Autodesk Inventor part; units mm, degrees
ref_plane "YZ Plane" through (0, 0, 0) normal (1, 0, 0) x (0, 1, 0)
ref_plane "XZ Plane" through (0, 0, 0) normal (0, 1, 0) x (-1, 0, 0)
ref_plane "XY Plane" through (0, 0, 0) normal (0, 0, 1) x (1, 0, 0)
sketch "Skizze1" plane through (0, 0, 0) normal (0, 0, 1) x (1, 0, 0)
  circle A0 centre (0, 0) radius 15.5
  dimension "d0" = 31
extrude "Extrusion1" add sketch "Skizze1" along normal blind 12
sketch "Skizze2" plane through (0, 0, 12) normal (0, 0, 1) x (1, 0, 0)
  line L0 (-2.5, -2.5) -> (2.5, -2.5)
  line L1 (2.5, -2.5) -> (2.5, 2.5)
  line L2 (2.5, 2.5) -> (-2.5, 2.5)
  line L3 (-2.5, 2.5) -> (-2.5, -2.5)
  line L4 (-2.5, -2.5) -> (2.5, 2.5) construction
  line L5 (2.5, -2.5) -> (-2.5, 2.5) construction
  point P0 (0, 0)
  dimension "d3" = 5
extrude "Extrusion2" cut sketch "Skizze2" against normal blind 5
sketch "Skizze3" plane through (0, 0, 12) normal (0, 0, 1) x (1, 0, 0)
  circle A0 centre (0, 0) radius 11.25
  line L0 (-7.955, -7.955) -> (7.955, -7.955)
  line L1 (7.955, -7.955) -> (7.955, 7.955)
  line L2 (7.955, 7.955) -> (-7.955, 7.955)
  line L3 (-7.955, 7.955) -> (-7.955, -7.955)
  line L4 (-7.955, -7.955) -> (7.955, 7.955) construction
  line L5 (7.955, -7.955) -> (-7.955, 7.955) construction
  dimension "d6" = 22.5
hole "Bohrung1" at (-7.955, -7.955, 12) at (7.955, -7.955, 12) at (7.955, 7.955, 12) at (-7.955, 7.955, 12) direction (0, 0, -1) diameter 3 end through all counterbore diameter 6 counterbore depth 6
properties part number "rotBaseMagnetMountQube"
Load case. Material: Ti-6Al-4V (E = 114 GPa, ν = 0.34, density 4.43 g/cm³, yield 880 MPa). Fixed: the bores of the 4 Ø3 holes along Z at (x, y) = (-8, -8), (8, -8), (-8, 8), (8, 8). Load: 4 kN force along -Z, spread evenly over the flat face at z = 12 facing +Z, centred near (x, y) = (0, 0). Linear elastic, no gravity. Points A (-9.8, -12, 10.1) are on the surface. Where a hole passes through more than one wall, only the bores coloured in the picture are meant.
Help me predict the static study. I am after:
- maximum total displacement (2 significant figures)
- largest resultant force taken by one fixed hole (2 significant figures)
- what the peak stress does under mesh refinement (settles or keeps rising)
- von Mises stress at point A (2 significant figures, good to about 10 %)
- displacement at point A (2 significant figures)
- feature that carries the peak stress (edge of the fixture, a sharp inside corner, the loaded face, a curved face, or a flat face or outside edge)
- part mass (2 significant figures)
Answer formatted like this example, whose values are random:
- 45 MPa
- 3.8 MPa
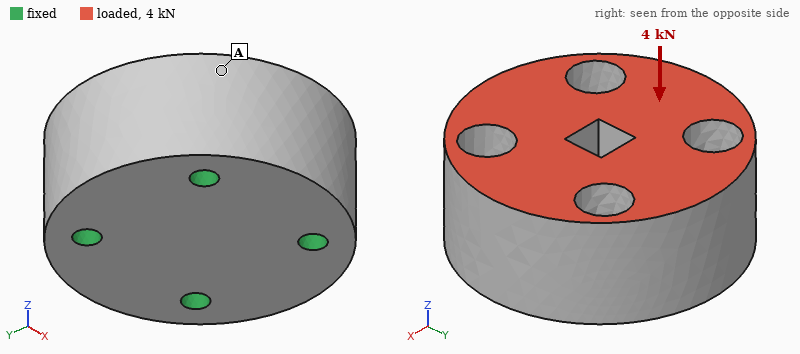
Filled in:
- 1.7 µm
- 1.0 kN
- keeps rising
- 9.1 MPa
- 1.0 µm
- edge of the fixture
- 36 g
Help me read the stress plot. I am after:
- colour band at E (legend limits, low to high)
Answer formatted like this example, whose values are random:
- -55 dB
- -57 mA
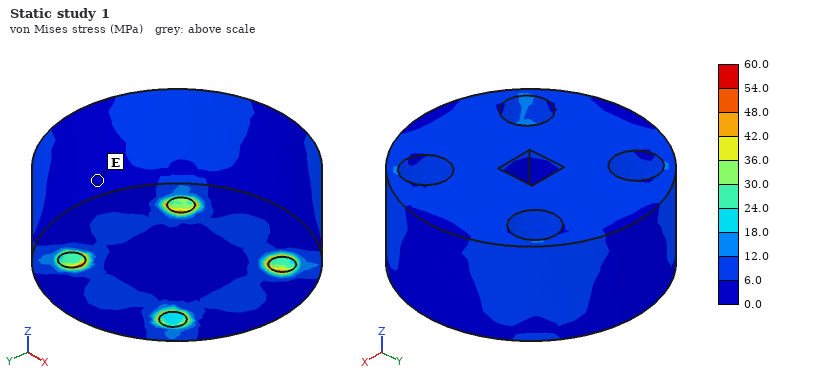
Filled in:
- 0.0 to 6.0 MPa
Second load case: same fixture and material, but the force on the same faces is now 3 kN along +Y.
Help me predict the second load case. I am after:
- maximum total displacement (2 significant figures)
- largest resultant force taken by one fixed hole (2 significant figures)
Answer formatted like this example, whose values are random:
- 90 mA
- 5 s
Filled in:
- 4.1 µm
- 1.0 kN
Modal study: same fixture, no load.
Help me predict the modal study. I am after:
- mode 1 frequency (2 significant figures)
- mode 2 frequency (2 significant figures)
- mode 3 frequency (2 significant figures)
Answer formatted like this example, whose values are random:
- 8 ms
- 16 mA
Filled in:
- 45 kHz
- 45 kHz
- 51 kHz
